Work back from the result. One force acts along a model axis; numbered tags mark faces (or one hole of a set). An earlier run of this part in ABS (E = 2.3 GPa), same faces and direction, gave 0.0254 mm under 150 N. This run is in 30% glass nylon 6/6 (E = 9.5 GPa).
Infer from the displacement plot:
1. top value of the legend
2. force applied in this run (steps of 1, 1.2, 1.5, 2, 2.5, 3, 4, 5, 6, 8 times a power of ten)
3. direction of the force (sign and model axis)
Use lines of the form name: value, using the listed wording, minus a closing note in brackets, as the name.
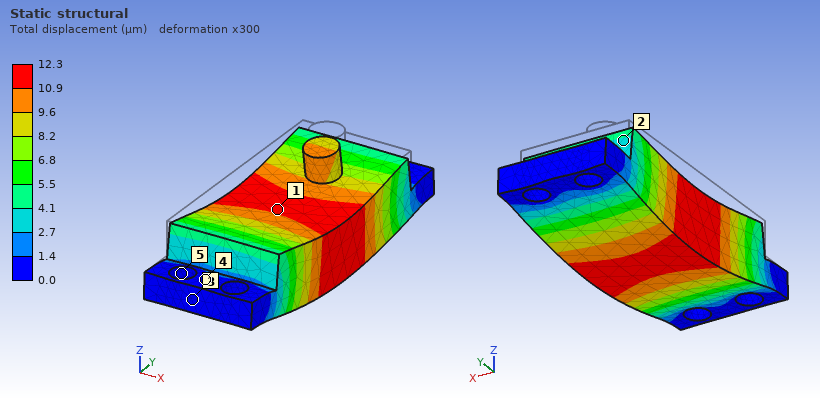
top value of the legend: 12.3 µm
force applied in this run: 300 N
direction of the force: -Z
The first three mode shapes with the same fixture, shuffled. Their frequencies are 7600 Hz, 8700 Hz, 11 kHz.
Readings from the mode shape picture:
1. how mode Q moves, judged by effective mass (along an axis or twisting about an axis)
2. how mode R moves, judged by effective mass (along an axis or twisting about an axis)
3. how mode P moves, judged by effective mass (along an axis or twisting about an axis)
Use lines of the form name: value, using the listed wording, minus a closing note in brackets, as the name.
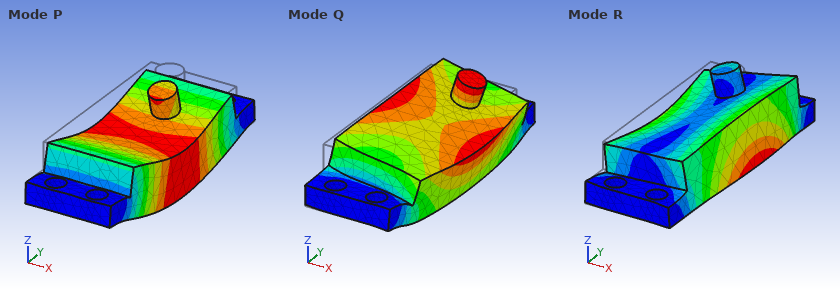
how mode Q moves, judged by effective mass: along X
how mode R moves, judged by effective mass: along X
how mode P moves, judged by effective mass: along Z
